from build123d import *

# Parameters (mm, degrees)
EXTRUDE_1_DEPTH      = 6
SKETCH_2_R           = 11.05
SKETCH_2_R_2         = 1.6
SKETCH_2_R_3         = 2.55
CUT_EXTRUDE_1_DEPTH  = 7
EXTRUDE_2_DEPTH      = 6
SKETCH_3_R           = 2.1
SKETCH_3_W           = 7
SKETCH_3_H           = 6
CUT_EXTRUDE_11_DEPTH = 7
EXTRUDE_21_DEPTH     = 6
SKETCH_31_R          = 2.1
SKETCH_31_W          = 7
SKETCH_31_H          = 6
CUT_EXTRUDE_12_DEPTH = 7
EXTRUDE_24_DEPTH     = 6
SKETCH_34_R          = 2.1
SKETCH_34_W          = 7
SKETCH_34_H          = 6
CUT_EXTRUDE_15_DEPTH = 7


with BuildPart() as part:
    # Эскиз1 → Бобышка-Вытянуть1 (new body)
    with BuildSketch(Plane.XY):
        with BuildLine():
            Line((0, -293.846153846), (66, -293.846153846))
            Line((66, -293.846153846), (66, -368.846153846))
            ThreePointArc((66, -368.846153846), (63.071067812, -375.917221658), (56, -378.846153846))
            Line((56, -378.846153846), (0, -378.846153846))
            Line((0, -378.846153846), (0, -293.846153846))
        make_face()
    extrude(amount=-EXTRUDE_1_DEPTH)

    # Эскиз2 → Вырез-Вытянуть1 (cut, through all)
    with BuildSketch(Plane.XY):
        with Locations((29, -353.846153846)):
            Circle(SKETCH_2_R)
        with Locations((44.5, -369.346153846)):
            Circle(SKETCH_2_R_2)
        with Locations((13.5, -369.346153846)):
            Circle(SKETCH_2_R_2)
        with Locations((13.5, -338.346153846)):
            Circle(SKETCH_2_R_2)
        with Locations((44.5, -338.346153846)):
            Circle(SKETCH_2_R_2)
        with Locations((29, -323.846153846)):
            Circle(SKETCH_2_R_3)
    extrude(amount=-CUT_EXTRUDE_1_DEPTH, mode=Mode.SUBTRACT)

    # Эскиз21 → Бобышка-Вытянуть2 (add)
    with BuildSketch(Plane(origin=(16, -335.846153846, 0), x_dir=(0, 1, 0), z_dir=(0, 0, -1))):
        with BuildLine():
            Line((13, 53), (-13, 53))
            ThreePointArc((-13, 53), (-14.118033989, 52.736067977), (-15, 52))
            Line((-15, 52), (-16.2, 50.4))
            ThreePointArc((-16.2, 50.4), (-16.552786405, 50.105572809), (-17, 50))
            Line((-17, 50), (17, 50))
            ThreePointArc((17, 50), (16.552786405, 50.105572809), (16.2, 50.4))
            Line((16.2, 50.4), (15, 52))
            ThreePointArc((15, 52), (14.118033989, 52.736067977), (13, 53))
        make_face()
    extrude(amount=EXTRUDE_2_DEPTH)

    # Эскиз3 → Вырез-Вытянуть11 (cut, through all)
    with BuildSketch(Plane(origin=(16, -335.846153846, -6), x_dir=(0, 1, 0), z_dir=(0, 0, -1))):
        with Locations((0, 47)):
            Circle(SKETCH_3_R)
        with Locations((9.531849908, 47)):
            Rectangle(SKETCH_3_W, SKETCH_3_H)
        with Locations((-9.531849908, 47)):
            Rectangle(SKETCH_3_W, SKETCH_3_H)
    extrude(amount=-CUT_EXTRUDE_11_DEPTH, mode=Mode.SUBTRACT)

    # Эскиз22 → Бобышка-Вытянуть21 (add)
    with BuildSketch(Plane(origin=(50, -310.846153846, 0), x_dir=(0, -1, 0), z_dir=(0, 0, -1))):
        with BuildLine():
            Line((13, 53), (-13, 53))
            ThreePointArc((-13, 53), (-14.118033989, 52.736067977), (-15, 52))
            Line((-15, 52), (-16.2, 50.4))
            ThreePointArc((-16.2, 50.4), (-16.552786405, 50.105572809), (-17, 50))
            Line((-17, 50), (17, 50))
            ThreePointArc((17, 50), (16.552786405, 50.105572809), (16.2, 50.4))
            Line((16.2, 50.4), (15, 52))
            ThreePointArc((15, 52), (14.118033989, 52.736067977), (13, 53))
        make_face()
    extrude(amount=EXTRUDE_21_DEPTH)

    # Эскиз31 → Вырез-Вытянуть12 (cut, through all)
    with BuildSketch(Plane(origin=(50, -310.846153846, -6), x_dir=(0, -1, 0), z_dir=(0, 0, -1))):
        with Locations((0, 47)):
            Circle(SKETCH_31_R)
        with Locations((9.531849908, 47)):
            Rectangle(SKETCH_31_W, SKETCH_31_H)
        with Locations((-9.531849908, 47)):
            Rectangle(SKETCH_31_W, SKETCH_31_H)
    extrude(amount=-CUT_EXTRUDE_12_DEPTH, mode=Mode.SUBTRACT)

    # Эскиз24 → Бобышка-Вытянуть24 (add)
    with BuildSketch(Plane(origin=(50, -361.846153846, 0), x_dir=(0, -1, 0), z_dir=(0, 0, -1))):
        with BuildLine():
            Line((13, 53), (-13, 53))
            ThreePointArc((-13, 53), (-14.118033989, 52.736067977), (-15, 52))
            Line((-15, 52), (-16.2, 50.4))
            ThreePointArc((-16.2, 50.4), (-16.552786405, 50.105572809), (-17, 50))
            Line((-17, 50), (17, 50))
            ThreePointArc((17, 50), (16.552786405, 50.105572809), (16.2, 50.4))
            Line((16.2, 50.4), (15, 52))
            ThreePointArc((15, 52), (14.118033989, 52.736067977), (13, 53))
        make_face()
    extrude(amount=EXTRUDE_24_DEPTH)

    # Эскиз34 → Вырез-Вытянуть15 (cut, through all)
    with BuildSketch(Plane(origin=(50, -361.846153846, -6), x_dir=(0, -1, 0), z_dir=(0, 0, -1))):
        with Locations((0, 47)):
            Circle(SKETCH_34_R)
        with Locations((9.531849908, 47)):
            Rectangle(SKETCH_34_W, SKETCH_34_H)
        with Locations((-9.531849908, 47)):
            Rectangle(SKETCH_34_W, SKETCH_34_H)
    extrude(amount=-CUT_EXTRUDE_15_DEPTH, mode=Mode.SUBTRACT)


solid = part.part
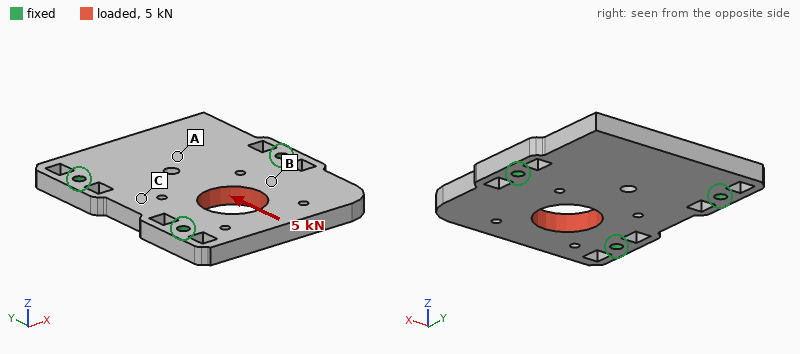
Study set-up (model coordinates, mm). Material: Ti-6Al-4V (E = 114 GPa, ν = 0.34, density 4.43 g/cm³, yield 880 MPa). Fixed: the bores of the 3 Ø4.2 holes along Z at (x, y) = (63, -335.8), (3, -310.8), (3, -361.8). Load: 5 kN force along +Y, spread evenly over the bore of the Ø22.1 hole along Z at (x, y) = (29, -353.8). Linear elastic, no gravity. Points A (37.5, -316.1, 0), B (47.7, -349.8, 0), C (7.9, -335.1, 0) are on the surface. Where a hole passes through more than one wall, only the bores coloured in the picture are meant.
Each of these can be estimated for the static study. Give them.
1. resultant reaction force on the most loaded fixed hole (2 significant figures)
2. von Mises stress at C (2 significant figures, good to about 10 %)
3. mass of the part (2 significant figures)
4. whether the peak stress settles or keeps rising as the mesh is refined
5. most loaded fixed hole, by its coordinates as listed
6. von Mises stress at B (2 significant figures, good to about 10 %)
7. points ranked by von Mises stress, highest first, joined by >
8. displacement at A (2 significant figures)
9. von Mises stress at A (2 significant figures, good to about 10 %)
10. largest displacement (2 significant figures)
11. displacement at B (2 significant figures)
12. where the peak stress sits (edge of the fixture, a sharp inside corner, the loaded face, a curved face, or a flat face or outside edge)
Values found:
2.1 kN
9.6 MPa
140 g
keeps rising
(63, -335.8)
16 MPa
B > C > A
4.1 µm
5.1 MPa
9.5 µm
5.2 µm
edge of the fixture
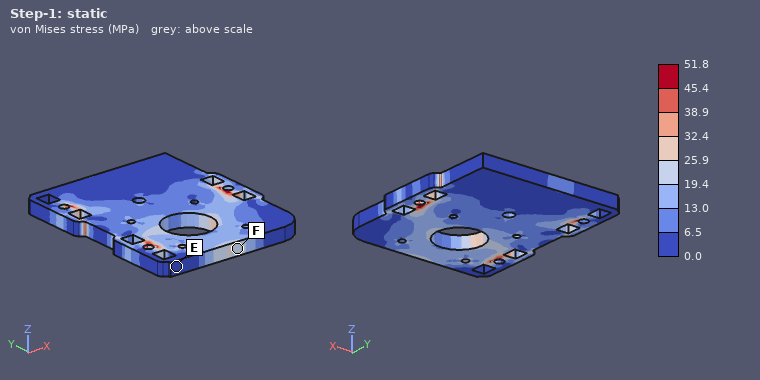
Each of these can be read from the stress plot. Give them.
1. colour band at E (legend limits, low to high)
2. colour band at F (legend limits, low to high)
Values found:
0.0 to 6.5 MPa
19.4 to 25.9 MPa
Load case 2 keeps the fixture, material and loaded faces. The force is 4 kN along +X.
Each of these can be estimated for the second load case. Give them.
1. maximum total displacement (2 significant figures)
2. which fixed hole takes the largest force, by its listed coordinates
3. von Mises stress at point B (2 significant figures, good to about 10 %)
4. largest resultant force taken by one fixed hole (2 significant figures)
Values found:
6.0 µm
(3, -361.8)
11 MPa
2.0 kN
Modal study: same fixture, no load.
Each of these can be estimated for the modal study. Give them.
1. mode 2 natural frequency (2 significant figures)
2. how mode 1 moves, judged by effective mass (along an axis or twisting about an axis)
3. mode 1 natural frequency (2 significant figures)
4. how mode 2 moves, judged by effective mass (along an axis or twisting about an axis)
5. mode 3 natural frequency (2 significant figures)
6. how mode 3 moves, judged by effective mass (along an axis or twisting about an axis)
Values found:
3400 Hz
twisting about X
2900 Hz
along Z
6800 Hz
along Z
